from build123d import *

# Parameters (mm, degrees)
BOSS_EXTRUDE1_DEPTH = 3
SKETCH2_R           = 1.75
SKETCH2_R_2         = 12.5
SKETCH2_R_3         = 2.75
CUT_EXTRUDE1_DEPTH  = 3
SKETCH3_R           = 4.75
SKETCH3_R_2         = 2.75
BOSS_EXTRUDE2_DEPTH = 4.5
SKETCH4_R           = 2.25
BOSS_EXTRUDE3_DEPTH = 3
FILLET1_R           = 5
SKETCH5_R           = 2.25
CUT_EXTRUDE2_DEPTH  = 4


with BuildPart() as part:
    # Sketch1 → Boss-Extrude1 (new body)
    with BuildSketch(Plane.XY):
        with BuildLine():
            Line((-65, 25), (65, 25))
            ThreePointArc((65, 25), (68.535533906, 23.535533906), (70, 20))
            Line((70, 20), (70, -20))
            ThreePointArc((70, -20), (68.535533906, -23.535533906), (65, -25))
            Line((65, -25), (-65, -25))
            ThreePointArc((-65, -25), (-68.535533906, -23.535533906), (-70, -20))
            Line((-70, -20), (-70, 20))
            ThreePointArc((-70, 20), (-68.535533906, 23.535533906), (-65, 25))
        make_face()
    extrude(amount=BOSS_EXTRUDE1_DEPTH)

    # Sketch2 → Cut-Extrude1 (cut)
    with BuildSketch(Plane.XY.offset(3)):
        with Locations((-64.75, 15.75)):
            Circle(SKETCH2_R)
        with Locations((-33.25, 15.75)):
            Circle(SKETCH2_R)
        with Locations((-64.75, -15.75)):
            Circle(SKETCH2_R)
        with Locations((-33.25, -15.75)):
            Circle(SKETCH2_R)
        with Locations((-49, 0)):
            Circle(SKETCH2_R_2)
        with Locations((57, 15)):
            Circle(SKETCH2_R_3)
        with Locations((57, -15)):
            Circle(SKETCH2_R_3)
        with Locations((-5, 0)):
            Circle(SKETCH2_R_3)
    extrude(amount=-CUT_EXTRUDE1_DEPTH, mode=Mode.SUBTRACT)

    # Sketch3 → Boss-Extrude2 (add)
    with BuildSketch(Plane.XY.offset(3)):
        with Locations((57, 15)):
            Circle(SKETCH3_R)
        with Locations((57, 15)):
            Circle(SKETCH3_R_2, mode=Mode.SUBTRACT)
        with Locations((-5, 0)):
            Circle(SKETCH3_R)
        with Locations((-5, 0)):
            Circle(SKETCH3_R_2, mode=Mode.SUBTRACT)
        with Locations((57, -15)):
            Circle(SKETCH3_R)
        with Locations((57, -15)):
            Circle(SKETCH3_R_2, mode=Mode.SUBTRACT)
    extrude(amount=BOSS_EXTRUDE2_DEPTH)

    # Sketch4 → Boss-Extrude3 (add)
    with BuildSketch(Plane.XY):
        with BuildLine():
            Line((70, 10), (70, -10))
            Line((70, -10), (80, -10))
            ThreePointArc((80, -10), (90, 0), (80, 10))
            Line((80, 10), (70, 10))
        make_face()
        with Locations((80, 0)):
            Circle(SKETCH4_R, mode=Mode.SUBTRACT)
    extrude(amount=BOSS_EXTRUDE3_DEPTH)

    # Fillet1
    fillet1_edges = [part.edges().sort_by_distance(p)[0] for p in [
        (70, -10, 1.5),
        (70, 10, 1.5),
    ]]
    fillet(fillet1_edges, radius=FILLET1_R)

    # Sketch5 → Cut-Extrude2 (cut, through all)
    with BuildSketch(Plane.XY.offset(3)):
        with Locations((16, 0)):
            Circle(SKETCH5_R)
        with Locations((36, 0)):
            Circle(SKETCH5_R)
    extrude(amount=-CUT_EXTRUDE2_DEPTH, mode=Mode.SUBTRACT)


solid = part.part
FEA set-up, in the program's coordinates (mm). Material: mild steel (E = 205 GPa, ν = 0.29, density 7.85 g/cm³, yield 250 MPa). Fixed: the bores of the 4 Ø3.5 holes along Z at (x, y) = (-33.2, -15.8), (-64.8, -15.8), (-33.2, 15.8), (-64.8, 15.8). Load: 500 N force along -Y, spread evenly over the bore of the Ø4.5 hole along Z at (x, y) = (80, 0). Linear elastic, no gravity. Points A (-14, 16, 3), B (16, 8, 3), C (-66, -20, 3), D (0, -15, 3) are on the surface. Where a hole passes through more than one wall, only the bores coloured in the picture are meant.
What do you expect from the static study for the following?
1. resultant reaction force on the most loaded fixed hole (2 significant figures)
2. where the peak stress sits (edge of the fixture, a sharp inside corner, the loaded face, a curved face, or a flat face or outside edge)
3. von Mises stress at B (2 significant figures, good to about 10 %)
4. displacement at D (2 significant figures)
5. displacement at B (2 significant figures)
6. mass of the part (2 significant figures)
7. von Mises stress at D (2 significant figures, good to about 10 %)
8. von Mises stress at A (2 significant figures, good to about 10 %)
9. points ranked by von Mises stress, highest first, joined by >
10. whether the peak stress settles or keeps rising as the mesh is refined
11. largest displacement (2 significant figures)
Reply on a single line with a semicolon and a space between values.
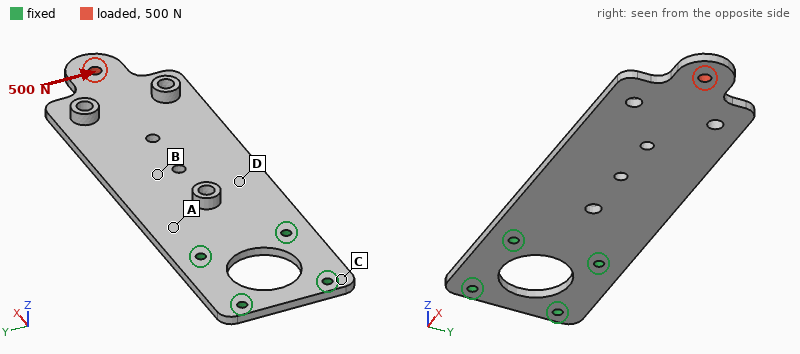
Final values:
1.5 kN; edge of the fixture; 12 MPa; 8.9 µm; 14 µm; 160 g; 19 MPa; 26 MPa; A > D > B > C; keeps rising; 56 µm
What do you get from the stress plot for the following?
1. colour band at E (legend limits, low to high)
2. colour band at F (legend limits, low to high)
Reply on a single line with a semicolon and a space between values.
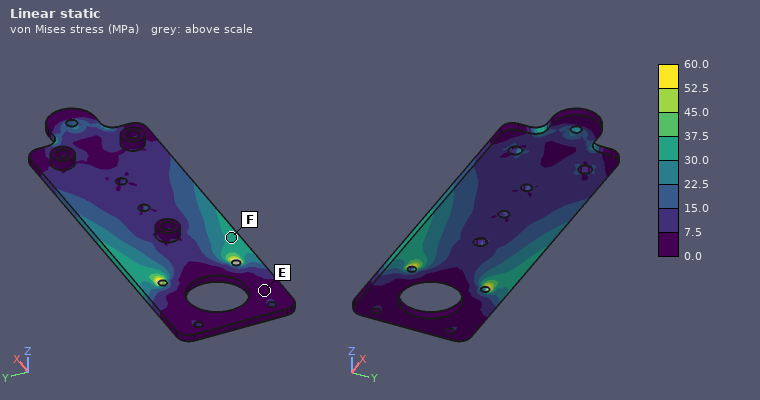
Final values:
0.0 to 7.5 MPa; 30.0 to 37.5 MPa
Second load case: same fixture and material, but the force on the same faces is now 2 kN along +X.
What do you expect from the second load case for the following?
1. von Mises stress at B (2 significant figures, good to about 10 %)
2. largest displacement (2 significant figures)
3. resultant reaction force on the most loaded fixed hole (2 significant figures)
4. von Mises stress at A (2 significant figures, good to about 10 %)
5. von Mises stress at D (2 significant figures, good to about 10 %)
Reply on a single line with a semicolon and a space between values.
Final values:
13 MPa; 13 µm; 940 N; 15 MPa; 13 MPa
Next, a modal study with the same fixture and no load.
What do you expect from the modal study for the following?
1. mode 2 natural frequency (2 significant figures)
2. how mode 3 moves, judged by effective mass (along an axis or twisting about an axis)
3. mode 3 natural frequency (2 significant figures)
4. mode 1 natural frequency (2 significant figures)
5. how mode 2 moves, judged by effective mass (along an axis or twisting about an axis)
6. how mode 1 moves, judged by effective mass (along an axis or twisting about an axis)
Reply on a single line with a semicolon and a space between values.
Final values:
1000 Hz; along Z; 1200 Hz; 200 Hz; twisting about X; along Z
